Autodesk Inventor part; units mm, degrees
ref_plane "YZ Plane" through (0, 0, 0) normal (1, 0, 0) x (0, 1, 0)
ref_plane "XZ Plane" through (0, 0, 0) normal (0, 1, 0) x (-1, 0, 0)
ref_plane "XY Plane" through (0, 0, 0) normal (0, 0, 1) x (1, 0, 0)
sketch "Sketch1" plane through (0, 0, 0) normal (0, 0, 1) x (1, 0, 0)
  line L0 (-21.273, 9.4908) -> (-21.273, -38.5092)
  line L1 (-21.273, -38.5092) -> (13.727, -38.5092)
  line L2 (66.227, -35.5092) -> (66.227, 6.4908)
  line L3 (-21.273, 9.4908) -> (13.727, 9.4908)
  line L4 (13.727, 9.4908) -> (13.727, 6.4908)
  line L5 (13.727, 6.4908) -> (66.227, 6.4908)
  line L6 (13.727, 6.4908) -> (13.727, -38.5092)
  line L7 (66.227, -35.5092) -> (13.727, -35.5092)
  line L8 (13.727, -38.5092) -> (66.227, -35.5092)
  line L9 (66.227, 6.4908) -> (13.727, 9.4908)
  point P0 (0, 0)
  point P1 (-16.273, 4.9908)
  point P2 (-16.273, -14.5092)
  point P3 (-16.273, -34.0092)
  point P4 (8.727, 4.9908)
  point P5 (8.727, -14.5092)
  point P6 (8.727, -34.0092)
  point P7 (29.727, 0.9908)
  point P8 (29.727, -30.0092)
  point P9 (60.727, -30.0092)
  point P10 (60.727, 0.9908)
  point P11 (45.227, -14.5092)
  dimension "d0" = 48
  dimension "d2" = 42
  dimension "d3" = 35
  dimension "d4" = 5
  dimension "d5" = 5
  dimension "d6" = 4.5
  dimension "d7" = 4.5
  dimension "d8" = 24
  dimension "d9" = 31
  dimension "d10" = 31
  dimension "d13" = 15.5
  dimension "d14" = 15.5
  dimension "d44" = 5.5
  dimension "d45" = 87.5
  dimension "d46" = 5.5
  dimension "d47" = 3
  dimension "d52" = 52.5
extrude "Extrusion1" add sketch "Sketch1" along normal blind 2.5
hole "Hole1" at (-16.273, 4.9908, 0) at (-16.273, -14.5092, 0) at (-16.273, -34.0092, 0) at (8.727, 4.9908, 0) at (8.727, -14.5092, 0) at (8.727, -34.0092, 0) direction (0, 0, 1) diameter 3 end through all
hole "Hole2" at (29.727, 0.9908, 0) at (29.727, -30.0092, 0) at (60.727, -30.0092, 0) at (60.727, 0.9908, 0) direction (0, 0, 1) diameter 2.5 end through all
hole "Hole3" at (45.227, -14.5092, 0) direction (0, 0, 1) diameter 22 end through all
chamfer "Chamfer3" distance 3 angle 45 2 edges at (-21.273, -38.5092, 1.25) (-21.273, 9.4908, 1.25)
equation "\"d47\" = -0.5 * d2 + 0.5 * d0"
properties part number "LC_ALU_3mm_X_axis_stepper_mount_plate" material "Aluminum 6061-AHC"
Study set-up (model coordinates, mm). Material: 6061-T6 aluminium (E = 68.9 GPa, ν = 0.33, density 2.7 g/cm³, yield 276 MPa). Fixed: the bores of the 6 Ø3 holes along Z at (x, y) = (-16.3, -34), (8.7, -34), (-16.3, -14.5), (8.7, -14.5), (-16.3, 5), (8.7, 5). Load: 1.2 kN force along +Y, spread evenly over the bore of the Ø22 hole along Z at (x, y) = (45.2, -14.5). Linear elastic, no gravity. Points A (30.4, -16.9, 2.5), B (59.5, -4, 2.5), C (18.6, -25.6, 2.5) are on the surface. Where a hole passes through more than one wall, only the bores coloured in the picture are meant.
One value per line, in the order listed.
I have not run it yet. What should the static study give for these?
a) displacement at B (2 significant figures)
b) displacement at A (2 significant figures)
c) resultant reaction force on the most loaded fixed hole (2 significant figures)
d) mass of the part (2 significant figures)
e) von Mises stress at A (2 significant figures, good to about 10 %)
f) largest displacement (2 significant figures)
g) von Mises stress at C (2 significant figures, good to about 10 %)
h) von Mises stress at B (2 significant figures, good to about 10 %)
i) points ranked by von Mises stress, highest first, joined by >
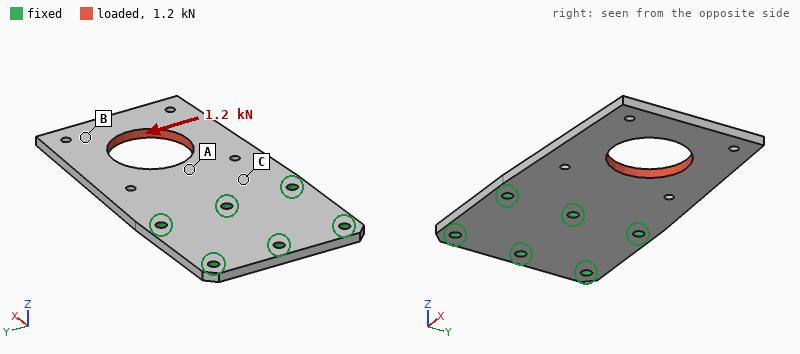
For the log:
61 µm
16 µm
1.1 kN
24 g
38 MPa
68 µm
22 MPa
7.2 MPa
A > C > B
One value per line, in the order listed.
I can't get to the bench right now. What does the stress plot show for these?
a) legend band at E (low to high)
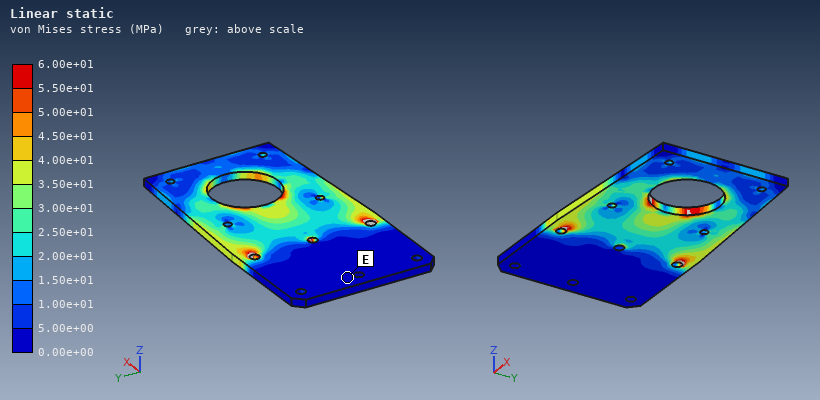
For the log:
0.00e+00 to 5.00e+00 MPa
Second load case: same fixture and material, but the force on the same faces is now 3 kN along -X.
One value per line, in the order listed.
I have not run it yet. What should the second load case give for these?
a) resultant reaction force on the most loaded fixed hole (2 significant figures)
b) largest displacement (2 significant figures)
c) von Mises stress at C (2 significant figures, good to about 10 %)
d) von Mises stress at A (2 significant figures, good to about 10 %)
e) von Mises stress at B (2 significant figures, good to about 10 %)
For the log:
900 N
35 µm
21 MPa
22 MPa
22 MPa
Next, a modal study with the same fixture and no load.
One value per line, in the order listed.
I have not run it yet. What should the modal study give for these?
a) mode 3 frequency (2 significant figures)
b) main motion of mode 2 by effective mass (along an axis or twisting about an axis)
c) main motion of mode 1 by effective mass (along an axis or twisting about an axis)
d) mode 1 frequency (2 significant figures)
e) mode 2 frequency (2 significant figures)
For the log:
3600 Hz
twisting about X
along Z
690 Hz
1800 Hz
